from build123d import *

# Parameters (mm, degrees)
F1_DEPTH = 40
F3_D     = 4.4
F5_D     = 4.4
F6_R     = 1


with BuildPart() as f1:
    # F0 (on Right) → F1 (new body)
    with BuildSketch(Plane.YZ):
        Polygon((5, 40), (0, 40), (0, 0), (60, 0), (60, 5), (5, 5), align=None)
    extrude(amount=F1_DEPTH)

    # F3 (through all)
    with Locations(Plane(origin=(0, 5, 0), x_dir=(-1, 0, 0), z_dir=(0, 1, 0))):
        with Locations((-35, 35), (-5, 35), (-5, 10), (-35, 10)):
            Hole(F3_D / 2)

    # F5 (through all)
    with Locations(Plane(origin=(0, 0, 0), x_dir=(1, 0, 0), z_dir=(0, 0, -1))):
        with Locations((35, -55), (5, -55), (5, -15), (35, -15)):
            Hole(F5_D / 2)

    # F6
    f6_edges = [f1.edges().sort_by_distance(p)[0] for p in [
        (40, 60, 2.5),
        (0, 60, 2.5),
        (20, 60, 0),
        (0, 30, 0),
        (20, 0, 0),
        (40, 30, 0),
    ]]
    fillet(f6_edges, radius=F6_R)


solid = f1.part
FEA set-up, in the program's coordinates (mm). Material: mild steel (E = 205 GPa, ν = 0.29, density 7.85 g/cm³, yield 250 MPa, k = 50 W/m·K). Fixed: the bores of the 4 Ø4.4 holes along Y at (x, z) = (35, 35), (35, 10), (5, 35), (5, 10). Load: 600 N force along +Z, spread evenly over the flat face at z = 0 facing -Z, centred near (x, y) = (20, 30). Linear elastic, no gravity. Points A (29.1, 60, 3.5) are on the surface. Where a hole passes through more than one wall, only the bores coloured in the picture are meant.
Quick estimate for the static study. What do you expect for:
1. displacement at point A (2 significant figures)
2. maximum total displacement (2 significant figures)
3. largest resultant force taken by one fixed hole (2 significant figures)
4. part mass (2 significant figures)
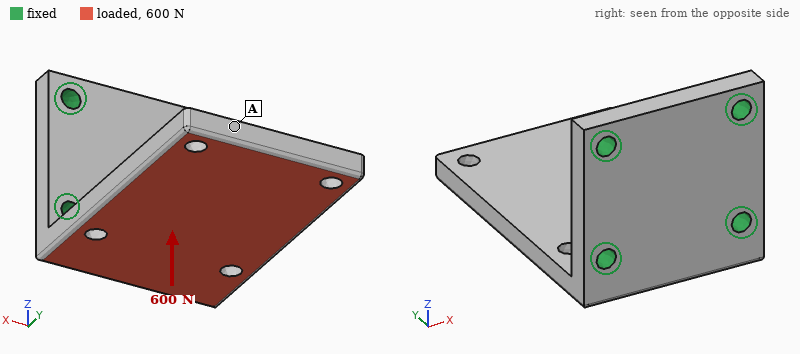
0.23 mm
0.23 mm
240 N
140 g
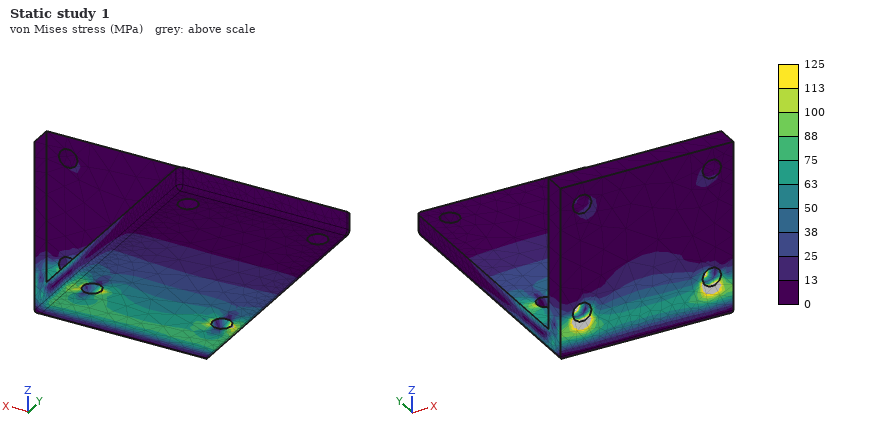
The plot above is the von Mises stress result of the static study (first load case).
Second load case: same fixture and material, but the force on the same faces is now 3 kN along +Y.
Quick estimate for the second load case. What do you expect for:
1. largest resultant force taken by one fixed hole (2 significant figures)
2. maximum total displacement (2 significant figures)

1.6 kN
0.19 mm
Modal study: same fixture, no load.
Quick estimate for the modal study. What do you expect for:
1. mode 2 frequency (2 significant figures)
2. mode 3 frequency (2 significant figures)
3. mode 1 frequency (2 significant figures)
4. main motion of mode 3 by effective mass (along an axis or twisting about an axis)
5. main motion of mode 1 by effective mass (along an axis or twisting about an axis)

3700 Hz
4900 Hz
1100 Hz
along X
along Z
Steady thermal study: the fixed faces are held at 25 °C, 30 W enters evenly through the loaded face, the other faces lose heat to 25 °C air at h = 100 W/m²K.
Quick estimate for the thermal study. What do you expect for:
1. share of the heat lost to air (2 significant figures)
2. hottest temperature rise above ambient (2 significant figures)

47 %
51 K
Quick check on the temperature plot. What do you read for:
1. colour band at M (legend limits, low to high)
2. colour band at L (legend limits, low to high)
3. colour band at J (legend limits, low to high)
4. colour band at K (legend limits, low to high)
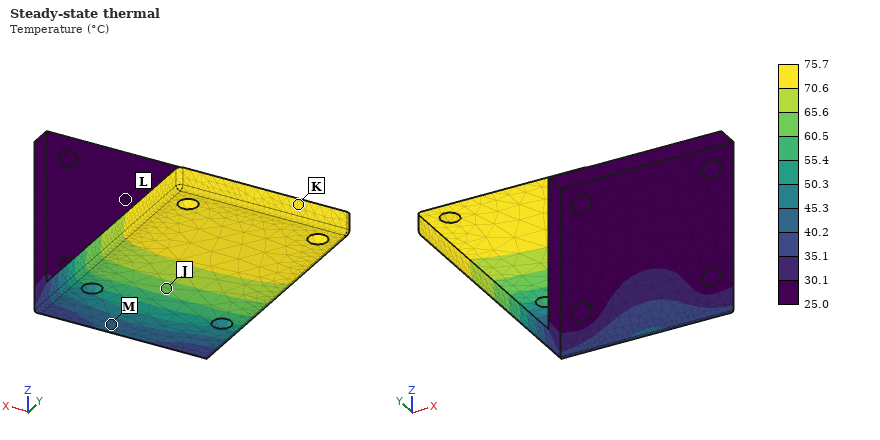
40.2 to 45.3 °C
25.0 to 30.1 °C
60.5 to 65.6 °C
70.6 to 75.7 °C
